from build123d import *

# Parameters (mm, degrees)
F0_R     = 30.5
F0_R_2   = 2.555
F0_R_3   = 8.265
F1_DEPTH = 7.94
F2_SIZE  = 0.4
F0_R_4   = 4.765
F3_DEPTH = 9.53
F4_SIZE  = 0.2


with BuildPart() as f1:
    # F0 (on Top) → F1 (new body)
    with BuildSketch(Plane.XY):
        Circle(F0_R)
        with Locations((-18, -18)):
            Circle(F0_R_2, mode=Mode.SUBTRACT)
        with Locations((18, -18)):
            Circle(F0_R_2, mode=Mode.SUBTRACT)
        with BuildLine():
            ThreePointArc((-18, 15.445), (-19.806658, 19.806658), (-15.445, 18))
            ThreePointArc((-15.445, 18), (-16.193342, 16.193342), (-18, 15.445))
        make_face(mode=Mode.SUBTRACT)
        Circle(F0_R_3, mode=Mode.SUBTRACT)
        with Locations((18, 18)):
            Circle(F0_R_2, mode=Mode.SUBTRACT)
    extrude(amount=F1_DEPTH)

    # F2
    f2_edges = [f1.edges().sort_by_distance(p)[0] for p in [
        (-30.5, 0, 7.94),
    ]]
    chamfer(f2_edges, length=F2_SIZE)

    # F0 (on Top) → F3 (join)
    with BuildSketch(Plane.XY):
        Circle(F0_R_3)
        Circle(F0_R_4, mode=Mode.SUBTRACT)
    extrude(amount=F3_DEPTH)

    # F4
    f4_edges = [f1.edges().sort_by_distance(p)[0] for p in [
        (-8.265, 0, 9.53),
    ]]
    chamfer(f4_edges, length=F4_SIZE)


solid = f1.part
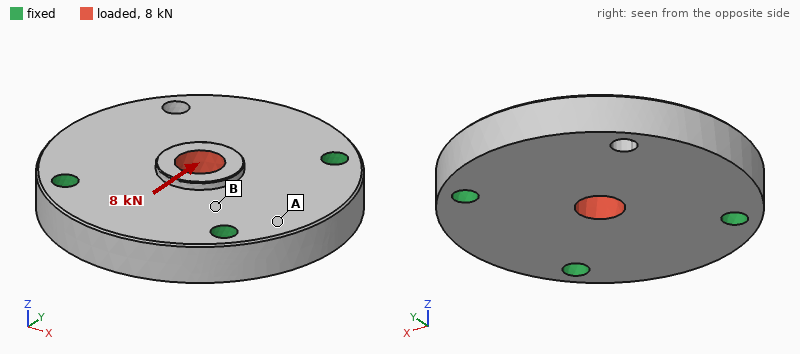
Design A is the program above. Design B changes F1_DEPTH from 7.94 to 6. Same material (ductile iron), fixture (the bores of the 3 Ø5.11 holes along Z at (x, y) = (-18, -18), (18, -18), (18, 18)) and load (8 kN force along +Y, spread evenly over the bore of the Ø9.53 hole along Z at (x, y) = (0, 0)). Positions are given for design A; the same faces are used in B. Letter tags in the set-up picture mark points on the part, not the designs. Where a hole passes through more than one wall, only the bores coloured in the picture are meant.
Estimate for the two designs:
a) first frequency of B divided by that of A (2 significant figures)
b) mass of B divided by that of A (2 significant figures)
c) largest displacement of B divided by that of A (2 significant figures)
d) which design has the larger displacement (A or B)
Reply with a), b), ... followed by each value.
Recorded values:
a) 0.80
b) 0.77
c) 2.3
d) B
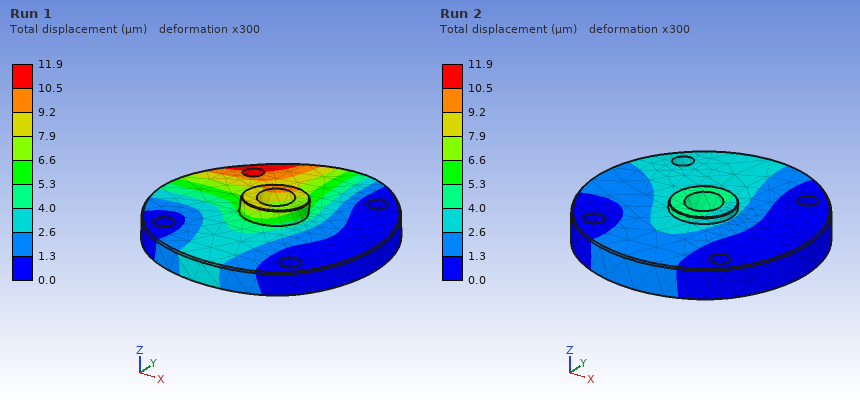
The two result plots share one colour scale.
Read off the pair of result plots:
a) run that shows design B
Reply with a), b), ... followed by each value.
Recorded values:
a) Run 1
